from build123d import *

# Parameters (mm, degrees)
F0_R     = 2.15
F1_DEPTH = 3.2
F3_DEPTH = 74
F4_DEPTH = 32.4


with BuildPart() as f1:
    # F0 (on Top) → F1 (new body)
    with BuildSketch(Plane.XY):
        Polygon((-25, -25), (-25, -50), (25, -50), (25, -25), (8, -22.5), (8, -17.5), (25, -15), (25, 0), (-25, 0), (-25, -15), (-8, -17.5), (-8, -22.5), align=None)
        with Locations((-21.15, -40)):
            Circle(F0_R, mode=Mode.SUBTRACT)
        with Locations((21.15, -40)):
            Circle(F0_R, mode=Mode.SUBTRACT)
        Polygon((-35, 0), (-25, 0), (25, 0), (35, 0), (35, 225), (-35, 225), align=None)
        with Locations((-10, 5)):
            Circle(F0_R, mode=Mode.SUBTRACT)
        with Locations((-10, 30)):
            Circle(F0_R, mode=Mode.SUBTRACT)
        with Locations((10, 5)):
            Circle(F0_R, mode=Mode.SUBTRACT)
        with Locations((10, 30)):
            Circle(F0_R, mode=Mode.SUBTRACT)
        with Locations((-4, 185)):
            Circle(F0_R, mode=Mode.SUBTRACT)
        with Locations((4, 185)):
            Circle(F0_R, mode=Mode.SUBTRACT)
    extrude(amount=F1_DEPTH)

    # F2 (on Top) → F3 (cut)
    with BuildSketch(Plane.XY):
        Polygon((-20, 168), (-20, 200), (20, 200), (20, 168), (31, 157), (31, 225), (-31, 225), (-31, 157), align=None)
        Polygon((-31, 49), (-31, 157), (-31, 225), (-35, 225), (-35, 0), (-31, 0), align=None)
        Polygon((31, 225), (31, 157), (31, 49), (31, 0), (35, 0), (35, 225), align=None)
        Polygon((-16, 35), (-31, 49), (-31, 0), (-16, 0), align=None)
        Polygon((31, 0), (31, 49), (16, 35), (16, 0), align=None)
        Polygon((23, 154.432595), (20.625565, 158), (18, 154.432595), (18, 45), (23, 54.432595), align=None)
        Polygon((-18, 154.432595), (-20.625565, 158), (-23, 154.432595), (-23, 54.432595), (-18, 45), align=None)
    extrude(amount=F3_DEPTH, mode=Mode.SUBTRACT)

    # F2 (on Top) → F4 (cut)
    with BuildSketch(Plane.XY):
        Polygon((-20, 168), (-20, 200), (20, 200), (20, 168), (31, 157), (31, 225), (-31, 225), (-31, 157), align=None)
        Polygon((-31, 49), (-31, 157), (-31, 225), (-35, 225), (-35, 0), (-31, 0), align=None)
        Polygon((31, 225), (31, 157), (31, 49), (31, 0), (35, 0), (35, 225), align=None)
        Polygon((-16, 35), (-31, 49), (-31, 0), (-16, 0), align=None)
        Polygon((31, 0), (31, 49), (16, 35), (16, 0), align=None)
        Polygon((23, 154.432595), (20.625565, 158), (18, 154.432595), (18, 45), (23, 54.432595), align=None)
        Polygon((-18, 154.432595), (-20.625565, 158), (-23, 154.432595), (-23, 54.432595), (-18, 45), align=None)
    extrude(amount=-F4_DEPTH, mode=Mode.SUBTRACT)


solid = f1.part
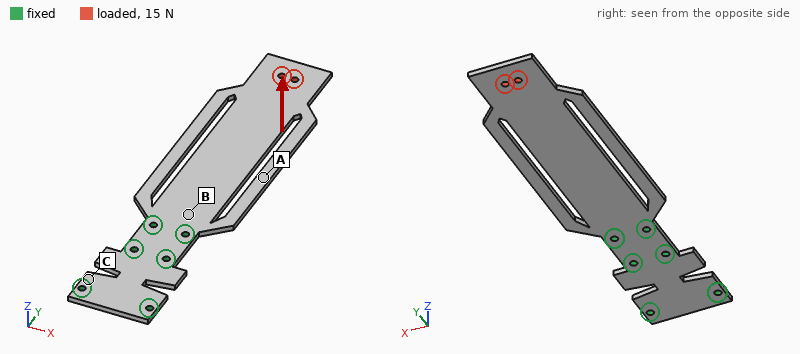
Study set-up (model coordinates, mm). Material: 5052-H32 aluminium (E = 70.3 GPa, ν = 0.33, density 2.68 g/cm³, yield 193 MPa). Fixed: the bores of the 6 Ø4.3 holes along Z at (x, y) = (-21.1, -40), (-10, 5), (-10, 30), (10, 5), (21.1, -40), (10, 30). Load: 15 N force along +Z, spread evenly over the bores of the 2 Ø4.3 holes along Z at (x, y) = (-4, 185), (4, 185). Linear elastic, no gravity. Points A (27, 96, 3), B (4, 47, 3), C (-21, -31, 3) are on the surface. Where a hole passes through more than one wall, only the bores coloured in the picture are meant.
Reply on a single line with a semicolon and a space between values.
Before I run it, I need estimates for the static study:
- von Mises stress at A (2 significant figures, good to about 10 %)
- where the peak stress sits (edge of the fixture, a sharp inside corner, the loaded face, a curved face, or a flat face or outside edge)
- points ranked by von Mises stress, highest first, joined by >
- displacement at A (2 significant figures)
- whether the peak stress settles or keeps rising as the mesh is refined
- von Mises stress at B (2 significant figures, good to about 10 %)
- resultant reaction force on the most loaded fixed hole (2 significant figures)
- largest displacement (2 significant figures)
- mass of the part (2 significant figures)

14 MPa; edge of the fixture; B > A > C; 0.50 mm; keeps rising; 24 MPa; 13 N; 2.3 mm; 98 g
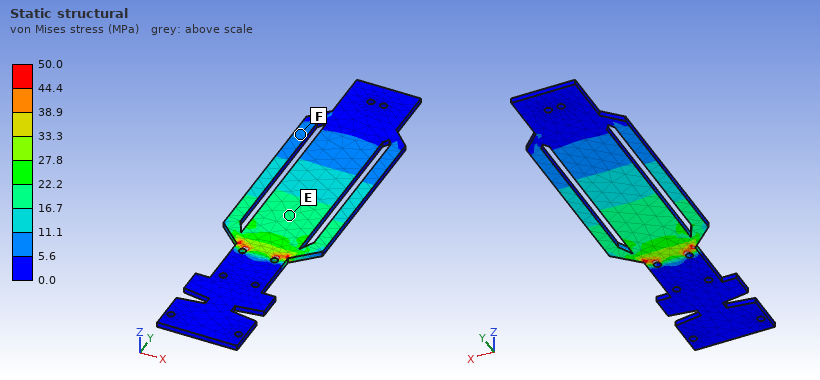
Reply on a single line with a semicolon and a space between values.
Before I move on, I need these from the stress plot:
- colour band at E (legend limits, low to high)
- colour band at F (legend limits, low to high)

16.7 to 22.2 MPa; 5.6 to 11.1 MPa
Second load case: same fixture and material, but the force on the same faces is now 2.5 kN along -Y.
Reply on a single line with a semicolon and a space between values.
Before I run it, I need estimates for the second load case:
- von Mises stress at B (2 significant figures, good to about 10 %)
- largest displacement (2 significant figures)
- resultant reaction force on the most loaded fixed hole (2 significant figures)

22 MPa; 50 µm; 1.1 kN
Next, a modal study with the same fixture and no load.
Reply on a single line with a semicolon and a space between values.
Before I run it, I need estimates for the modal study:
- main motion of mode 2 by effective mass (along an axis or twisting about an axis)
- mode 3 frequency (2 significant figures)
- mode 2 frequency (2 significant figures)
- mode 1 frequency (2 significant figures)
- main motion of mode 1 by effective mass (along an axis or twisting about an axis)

twisting about Y; 570 Hz; 530 Hz; 94 Hz; along Z
